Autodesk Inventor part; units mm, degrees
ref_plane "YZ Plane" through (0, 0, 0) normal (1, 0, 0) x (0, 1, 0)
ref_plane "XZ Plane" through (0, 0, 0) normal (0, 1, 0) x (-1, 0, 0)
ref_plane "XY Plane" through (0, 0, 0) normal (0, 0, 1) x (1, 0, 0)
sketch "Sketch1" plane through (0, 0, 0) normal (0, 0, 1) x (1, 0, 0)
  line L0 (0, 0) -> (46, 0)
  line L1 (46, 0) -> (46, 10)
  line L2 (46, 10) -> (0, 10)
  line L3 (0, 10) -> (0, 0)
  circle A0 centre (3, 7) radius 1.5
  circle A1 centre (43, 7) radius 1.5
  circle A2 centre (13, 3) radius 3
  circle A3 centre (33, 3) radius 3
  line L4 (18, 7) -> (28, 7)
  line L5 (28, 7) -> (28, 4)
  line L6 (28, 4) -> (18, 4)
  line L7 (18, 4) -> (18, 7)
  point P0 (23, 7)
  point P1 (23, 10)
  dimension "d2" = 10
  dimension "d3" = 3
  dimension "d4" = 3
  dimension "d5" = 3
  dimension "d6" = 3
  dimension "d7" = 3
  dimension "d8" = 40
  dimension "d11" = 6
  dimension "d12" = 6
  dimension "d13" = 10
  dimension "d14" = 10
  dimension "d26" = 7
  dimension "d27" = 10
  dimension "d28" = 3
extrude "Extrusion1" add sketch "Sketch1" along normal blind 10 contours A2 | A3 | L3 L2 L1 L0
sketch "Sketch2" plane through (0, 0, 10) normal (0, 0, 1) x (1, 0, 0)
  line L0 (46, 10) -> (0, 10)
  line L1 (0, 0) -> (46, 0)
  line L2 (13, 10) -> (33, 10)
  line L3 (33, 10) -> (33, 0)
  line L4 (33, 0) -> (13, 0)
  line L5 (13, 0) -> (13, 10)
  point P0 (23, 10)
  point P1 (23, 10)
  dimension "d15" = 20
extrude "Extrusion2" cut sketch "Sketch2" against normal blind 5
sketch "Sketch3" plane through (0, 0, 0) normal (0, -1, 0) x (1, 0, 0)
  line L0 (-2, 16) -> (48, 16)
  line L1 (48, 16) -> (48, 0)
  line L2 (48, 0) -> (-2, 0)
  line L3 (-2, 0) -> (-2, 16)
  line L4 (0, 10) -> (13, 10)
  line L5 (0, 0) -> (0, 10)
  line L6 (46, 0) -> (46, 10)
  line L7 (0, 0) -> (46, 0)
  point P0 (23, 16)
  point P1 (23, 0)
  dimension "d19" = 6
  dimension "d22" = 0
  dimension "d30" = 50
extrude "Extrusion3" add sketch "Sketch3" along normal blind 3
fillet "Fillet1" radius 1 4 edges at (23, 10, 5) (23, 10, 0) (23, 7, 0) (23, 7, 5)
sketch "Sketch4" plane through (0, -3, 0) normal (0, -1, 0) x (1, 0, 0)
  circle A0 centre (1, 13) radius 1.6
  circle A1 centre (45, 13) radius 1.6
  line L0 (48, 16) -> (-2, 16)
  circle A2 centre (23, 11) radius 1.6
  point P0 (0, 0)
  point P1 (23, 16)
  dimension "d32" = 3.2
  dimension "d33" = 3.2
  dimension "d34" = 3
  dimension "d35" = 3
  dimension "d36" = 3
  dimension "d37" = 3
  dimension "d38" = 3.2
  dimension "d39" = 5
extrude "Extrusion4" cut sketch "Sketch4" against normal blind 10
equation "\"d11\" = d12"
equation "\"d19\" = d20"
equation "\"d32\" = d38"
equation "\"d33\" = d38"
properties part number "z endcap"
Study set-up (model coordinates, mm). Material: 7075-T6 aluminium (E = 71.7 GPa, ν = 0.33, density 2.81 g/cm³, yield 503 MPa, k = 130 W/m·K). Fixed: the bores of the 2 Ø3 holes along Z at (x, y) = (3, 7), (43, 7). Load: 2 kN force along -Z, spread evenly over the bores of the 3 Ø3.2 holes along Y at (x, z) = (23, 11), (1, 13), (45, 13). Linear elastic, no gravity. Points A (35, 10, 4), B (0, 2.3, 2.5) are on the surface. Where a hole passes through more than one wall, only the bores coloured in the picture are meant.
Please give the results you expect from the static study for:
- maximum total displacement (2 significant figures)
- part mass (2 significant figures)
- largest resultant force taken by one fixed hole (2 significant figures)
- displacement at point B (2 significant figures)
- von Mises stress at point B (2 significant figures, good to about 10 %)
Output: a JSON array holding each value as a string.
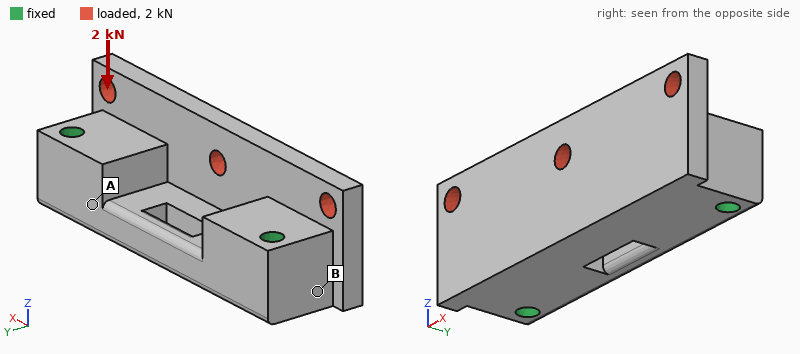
["18 µm", "16 g", "1.0 kN", "3.2 µm", "30 MPa"]
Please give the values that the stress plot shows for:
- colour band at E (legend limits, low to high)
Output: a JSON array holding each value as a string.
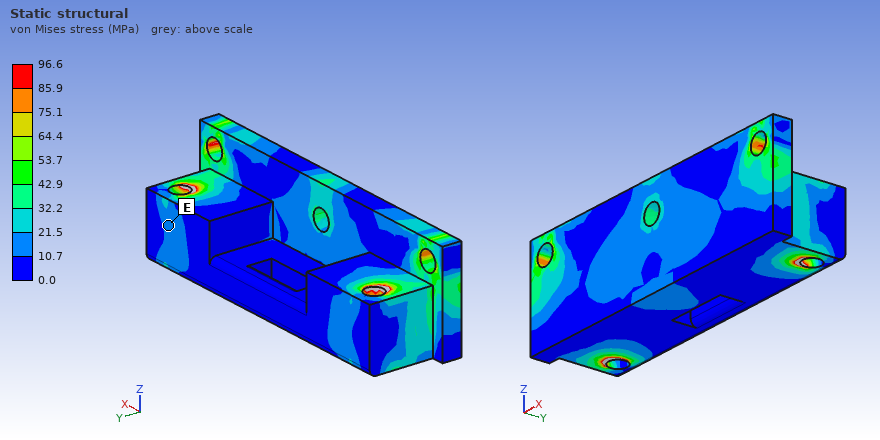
["10.7 to 21.5 MPa"]
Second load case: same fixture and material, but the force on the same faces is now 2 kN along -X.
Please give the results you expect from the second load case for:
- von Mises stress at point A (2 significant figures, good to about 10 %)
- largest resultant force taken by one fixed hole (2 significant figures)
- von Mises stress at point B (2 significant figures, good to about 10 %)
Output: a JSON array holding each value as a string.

["15 MPa", "1.1 kN", "23 MPa"]
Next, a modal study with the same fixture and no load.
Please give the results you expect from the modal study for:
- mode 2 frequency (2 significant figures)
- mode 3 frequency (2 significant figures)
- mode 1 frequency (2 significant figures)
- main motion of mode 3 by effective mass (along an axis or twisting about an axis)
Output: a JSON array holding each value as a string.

["23 kHz", "25 kHz", "18 kHz", "along X"]
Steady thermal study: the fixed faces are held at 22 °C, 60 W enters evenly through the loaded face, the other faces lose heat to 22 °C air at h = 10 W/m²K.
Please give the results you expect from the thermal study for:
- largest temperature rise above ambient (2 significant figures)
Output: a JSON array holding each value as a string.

["59 K"]
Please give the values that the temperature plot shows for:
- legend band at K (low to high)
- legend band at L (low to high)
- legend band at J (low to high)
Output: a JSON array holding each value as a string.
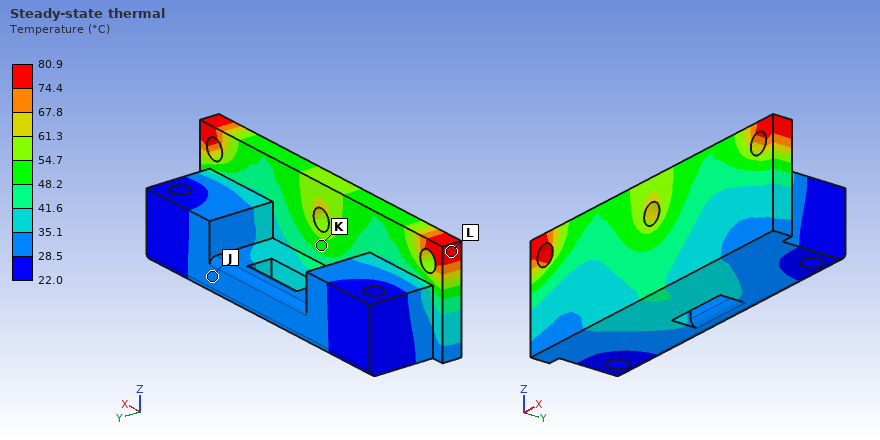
["48.2 to 54.7 °C", "74.4 to 80.9 °C", "28.5 to 35.1 °C"]
